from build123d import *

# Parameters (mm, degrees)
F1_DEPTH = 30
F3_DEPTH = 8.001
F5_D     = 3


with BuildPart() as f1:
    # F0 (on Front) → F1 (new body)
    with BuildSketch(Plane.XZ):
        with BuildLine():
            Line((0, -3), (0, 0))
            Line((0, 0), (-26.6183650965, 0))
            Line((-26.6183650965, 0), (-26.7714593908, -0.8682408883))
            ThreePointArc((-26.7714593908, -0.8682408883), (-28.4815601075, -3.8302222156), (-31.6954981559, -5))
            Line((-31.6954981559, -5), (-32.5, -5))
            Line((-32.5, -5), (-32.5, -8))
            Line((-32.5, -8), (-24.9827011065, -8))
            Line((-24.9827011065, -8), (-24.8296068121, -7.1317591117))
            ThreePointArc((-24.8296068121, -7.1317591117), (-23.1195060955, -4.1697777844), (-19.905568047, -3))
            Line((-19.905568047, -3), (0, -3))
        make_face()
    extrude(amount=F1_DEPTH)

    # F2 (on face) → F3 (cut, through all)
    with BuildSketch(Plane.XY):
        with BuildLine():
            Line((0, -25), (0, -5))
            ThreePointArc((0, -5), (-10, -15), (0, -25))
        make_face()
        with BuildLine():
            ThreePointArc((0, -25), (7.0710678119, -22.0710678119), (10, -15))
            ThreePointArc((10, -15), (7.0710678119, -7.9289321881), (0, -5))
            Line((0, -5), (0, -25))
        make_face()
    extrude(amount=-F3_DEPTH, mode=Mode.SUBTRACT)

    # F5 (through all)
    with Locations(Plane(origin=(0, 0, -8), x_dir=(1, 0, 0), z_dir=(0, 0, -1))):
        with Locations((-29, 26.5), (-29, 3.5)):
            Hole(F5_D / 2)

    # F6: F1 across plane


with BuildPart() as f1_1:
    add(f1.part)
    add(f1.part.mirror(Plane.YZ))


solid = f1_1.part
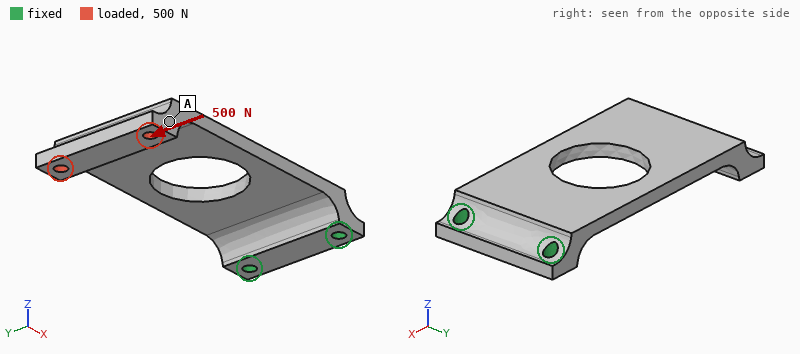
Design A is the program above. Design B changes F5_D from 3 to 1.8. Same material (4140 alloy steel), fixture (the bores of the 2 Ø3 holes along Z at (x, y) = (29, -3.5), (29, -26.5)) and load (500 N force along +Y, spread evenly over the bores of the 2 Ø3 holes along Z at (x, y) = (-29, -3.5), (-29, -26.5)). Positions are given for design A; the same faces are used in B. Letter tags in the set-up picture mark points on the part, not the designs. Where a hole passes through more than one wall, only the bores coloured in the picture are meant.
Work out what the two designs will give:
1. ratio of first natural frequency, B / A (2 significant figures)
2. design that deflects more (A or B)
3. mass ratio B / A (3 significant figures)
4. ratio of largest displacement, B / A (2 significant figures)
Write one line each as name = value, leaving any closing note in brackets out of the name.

ratio of first natural frequency, B / A = 0.97
design that deflects more = B
mass ratio B / A = 1.01
ratio of largest displacement, B / A = 1.1
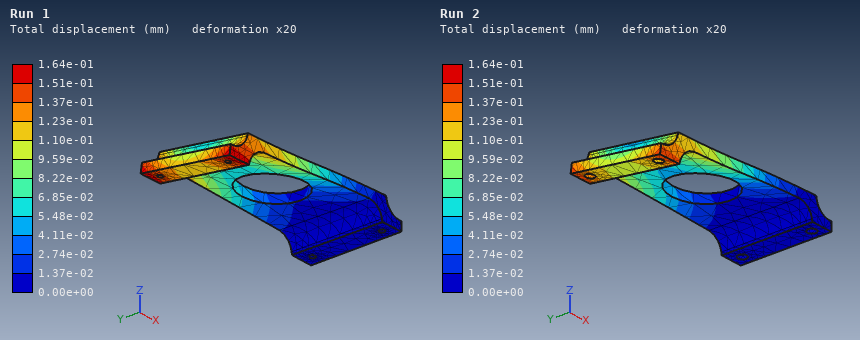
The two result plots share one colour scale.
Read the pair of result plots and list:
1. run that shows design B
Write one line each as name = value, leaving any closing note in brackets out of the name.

run that shows design B = Run 1
